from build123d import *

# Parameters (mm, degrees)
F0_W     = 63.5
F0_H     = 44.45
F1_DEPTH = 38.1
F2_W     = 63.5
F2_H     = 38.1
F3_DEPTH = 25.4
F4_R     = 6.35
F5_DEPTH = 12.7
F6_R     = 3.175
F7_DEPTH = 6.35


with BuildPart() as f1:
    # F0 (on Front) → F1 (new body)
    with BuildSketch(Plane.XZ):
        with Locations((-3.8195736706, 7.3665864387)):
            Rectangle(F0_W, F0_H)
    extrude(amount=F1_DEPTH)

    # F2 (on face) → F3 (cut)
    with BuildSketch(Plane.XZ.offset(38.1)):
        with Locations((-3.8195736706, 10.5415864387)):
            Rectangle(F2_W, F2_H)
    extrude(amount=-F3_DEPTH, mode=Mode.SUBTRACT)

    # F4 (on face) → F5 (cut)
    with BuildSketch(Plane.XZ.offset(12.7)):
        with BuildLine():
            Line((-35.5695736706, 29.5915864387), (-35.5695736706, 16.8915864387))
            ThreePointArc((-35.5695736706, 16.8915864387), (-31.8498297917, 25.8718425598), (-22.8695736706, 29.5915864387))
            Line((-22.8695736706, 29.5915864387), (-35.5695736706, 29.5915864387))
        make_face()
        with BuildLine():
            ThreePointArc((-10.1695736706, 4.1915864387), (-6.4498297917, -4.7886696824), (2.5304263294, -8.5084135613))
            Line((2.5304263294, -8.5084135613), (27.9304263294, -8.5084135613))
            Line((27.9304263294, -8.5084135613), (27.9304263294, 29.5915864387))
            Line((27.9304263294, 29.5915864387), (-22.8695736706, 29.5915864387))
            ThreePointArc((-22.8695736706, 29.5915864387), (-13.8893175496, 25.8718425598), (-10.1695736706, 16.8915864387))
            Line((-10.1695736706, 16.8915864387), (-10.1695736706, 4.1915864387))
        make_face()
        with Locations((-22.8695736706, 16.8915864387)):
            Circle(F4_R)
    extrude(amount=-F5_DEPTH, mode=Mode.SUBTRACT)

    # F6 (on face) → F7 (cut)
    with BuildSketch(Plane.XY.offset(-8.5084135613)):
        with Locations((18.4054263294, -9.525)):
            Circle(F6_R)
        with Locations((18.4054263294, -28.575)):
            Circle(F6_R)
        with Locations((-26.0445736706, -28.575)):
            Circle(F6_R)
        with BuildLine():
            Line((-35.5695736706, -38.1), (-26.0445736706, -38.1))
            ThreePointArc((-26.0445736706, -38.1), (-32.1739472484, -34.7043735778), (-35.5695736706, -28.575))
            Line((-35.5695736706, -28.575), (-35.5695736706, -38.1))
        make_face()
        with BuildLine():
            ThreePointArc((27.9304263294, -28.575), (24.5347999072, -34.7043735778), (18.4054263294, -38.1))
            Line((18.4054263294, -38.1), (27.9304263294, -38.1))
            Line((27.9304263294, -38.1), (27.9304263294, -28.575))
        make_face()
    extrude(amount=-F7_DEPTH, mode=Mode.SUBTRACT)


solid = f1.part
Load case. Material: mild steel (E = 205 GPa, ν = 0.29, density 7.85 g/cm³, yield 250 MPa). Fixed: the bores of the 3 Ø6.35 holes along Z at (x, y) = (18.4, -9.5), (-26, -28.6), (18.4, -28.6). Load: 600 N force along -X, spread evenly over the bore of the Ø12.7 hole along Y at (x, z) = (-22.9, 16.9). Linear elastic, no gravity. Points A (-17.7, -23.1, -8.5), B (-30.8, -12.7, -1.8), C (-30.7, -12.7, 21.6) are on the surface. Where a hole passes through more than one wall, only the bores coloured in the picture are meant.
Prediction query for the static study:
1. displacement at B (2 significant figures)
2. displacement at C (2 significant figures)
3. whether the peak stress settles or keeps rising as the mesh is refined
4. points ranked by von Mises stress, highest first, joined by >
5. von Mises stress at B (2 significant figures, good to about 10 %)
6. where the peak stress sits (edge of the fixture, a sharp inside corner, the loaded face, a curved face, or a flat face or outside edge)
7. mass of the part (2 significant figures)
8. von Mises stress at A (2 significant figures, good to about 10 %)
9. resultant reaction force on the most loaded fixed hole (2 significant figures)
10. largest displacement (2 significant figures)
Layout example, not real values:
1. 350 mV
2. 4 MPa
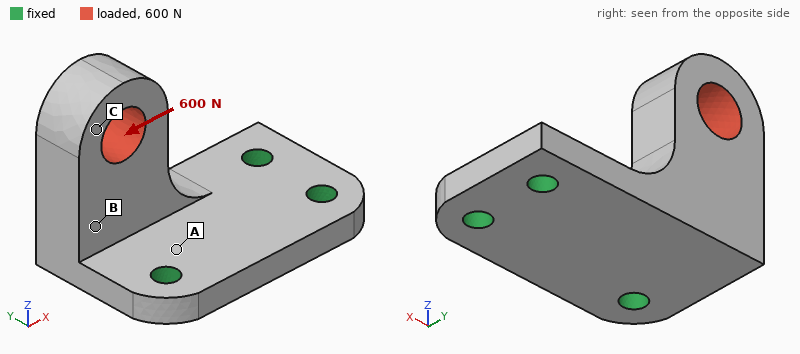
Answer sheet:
1. 8.5 µm
2. 19 µm
3. keeps rising
4. A > B > C
5. 7.8 MPa
6. edge of the fixture
7. 190 g
8. 16 MPa
9. 450 N
10. 23 µm
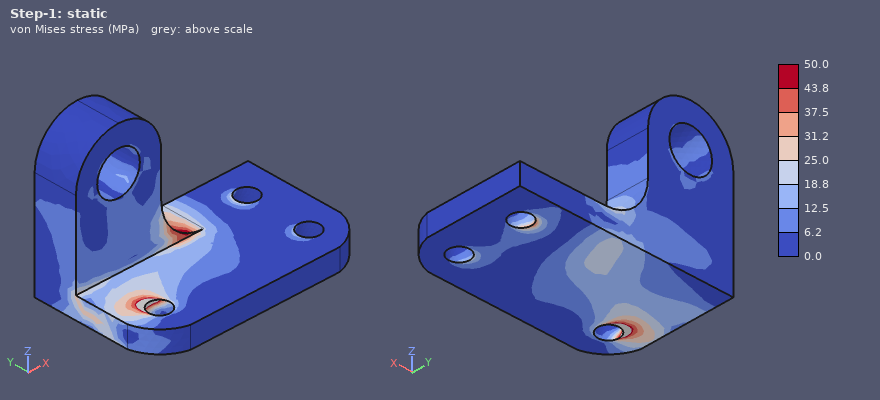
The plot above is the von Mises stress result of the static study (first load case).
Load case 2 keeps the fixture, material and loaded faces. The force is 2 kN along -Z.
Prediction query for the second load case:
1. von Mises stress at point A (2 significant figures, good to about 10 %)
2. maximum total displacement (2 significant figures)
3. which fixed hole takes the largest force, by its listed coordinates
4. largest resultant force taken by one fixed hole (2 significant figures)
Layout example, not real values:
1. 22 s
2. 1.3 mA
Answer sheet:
1. 58 MPa
2. 84 µm
3. (-26, -28.6)
4. 1.6 kN
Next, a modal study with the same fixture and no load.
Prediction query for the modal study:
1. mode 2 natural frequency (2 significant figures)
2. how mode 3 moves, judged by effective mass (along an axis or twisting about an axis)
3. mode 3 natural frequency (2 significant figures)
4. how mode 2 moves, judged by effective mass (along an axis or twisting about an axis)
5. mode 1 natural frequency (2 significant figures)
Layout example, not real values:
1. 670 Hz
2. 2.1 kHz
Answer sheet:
1. 5100 Hz
2. along Z
3. 7700 Hz
4. along X
5. 2400 Hz
